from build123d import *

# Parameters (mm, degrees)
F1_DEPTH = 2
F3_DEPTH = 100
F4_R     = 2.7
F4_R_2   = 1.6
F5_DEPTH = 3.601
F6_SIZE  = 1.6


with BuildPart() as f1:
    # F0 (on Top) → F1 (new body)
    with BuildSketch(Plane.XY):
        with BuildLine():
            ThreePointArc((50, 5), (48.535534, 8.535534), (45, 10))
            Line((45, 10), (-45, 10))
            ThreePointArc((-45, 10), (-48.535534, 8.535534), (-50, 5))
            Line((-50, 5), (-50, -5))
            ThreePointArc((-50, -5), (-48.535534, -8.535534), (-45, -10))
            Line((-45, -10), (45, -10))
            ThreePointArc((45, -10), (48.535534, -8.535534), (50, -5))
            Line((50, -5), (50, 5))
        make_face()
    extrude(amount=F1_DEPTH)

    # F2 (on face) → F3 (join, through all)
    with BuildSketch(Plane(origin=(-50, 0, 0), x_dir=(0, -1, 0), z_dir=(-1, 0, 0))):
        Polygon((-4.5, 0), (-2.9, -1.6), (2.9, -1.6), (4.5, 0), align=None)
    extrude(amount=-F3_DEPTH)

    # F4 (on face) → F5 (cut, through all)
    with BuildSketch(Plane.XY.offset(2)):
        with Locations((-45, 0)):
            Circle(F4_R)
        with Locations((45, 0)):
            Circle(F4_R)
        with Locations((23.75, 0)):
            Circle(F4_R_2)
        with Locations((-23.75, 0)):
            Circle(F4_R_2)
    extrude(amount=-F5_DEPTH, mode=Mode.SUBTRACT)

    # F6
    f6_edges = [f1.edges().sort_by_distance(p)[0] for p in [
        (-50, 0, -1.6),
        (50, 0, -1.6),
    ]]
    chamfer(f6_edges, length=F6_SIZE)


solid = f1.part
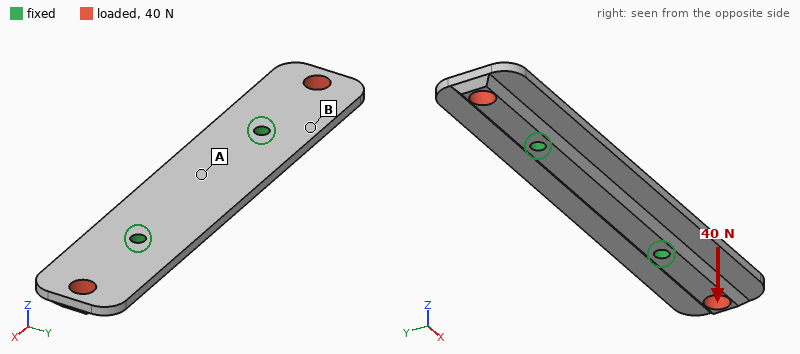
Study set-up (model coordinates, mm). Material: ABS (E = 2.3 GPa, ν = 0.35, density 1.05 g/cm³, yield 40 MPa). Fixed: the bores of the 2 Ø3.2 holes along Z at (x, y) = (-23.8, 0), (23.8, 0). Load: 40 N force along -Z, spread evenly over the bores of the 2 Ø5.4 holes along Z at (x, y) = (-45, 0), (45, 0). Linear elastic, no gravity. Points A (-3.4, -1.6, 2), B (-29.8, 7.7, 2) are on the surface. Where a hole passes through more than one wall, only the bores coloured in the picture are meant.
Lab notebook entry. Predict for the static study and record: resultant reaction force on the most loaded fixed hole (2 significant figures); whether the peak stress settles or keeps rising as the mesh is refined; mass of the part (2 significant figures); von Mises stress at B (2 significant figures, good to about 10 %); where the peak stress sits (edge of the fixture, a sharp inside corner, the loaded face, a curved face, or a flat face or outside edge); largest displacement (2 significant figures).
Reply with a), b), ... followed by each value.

a) 26 N
b) keeps rising
c) 5.1 g
d) 8.8 MPa
e) edge of the fixture
f) 0.86 mm
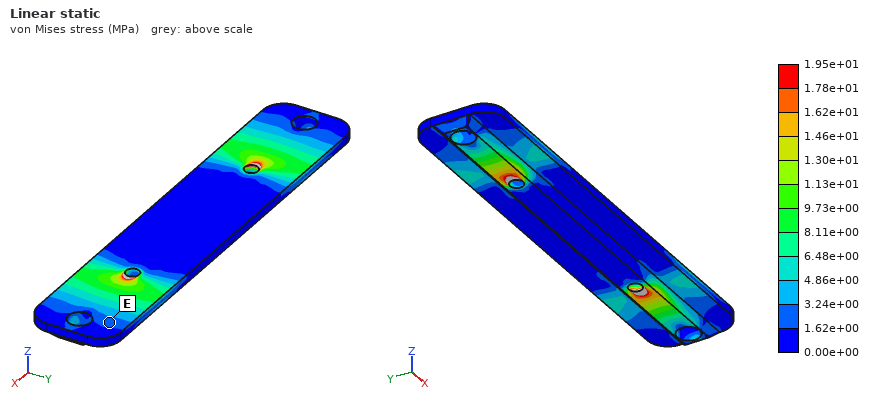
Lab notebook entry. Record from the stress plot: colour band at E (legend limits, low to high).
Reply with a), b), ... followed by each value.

a) 1.62e+00 to 3.24e+00 MPa
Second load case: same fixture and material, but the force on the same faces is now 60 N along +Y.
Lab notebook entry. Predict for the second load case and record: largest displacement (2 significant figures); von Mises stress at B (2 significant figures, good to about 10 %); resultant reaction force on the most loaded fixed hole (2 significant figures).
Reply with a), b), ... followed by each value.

a) 0.13 mm
b) 2.5 MPa
c) 30 N
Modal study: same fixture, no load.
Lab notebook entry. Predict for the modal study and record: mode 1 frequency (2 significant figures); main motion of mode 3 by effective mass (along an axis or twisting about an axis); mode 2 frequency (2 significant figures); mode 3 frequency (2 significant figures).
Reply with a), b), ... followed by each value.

a) 1300 Hz
b) along Z
c) 1300 Hz
d) 2100 Hz
